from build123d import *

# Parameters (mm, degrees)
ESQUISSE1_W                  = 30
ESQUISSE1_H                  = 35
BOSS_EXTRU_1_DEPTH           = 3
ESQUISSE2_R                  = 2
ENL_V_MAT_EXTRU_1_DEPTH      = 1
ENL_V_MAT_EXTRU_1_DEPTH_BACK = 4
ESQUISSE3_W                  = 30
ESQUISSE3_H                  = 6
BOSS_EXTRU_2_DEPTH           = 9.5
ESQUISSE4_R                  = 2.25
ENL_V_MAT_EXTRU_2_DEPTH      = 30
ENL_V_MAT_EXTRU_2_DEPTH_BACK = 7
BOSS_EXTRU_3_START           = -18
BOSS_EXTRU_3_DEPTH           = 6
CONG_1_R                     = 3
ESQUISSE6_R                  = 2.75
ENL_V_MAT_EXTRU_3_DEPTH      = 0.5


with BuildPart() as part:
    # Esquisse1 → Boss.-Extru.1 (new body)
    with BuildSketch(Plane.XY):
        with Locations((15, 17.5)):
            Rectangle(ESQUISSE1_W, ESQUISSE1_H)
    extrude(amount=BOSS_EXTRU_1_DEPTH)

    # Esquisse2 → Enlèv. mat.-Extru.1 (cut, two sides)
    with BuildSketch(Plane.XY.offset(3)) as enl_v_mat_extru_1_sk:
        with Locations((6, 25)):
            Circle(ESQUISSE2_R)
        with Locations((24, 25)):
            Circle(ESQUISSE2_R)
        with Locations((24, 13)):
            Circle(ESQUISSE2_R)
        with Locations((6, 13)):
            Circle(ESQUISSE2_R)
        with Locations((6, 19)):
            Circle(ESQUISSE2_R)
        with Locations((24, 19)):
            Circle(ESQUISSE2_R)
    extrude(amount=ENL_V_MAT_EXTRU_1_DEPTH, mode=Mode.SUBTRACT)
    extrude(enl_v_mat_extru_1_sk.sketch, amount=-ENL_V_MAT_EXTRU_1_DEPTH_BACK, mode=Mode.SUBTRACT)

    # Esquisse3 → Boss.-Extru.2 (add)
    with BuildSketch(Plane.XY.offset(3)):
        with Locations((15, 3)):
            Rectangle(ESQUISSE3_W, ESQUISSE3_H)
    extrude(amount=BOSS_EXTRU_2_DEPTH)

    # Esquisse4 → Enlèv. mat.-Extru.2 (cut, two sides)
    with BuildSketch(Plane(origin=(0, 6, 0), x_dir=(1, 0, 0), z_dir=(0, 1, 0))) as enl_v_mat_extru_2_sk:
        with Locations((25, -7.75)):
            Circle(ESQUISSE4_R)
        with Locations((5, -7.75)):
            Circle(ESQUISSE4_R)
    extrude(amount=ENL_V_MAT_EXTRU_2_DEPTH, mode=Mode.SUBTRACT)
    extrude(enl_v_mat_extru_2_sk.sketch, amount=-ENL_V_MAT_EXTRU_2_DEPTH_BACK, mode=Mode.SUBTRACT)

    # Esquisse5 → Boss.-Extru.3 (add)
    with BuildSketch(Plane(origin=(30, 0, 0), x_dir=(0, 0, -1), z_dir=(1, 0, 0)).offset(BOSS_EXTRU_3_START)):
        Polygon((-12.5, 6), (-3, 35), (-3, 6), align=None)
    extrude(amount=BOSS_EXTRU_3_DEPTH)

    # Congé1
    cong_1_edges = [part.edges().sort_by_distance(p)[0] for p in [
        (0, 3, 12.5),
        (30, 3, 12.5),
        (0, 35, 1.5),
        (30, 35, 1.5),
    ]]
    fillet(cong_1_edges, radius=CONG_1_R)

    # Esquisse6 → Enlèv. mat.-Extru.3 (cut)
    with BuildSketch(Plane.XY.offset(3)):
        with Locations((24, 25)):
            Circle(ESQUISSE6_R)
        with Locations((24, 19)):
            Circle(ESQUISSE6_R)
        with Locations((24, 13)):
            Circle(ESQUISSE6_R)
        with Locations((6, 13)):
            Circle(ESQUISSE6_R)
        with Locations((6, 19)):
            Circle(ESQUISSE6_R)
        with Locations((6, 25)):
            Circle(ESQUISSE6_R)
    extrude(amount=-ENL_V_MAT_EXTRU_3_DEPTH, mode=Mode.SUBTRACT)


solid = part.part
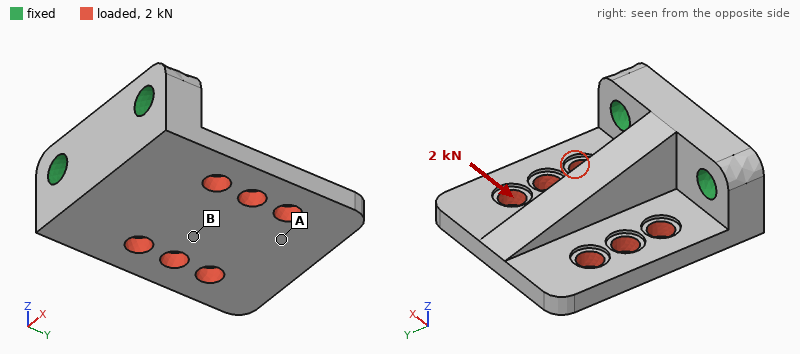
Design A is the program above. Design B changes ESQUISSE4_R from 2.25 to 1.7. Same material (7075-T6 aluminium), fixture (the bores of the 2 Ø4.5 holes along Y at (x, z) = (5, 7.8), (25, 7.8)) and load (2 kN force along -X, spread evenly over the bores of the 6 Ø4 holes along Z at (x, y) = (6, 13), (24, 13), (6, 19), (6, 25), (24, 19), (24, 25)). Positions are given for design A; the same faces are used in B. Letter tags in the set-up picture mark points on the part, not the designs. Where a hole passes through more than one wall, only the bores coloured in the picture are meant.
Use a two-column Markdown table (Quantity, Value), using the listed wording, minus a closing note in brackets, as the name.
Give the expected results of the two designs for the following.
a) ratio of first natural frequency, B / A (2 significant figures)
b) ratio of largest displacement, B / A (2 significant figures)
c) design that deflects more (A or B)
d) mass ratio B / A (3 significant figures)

| Quantity | Value |
|---|---|
| ratio of first natural frequency, B / A | 0.95 |
| ratio of largest displacement, B / A | 1.1 |
| design that deflects more | B |
| mass ratio B / A | 1.02 |
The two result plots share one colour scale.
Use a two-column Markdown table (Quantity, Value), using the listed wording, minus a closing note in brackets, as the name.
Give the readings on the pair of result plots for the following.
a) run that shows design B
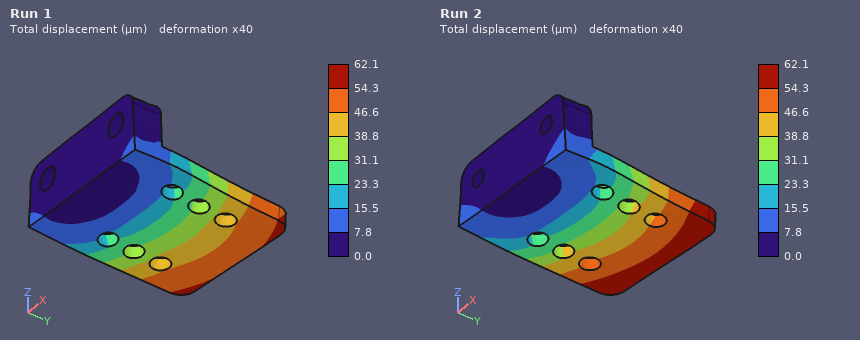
| Quantity | Value |
|---|---|
| run that shows design B | Run 2 |
